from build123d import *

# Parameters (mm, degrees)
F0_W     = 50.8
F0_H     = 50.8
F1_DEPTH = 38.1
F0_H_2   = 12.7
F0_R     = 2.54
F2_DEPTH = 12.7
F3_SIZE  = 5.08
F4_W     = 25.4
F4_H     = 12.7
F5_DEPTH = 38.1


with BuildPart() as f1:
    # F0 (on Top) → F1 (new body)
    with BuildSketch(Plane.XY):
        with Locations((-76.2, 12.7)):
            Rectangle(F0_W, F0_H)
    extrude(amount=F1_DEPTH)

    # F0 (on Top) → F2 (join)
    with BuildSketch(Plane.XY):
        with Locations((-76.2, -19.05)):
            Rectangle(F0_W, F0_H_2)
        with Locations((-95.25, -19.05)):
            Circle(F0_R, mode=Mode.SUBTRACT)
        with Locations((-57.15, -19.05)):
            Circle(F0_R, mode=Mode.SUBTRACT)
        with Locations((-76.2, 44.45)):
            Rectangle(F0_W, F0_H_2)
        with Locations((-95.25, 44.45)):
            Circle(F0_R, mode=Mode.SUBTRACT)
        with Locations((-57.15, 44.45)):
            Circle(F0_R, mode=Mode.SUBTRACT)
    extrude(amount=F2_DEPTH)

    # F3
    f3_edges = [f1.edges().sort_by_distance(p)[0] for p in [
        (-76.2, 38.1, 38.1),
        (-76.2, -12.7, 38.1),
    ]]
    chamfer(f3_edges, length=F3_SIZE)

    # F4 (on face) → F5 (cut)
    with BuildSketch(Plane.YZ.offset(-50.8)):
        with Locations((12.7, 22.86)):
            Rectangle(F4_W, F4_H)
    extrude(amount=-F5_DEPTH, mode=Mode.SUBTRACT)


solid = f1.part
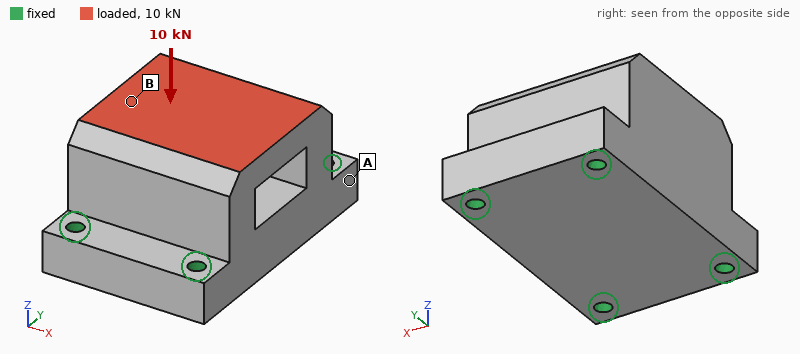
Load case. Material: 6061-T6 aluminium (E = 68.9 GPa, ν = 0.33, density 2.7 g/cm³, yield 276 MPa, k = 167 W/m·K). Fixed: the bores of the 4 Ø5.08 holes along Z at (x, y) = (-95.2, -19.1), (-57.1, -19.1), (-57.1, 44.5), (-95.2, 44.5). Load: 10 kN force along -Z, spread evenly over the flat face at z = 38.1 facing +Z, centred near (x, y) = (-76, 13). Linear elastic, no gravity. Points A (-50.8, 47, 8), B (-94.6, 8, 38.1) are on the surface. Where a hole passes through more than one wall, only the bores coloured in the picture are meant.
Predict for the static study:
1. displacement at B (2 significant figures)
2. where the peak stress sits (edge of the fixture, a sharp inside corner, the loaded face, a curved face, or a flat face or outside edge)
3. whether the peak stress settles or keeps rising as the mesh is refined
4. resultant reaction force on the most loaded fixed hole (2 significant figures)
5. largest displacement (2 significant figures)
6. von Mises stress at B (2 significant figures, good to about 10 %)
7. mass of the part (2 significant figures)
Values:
9.7 µm
edge of the fixture
keeps rising
2.7 kN
17 µm
7.8 MPa
270 g
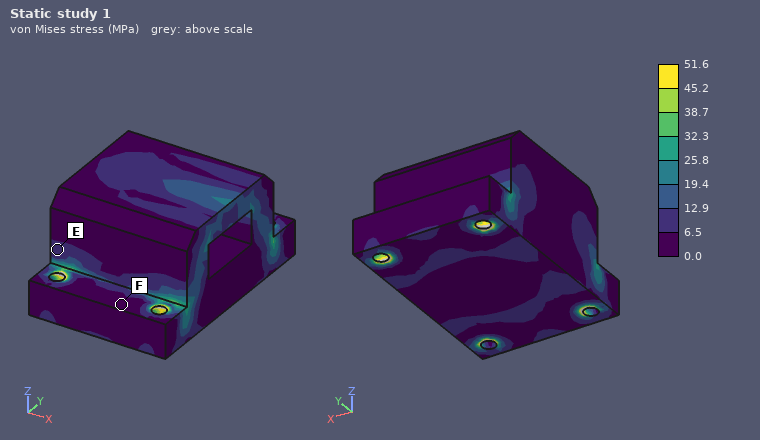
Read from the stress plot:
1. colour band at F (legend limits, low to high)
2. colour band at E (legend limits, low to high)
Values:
0.0 to 6.5 MPa
6.5 to 12.9 MPa
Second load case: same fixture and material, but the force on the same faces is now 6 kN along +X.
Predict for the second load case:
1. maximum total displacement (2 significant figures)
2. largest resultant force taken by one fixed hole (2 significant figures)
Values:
26 µm
3.0 kN
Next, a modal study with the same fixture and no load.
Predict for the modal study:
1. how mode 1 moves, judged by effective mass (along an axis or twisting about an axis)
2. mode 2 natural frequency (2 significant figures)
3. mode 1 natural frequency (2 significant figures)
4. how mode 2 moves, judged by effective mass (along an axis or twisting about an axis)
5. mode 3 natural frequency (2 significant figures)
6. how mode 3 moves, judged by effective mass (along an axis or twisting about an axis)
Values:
along X
11 kHz
9200 Hz
along Z
12 kHz
along Y
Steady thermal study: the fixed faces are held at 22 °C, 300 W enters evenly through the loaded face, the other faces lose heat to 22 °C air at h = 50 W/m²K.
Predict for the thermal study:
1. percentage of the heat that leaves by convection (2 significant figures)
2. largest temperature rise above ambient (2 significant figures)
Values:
6.5 %
59 K
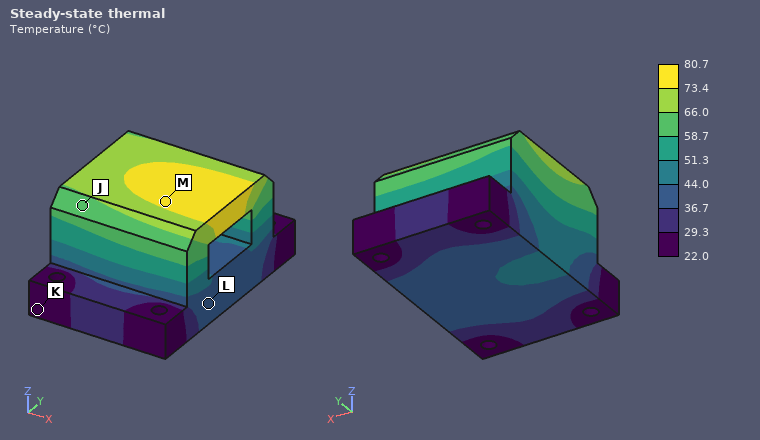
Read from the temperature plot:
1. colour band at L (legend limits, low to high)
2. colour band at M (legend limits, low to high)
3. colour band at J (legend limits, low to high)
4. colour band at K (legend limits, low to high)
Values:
36.7 to 44.0 °C
73.4 to 80.7 °C
58.7 to 66.0 °C
22.0 to 29.3 °C
